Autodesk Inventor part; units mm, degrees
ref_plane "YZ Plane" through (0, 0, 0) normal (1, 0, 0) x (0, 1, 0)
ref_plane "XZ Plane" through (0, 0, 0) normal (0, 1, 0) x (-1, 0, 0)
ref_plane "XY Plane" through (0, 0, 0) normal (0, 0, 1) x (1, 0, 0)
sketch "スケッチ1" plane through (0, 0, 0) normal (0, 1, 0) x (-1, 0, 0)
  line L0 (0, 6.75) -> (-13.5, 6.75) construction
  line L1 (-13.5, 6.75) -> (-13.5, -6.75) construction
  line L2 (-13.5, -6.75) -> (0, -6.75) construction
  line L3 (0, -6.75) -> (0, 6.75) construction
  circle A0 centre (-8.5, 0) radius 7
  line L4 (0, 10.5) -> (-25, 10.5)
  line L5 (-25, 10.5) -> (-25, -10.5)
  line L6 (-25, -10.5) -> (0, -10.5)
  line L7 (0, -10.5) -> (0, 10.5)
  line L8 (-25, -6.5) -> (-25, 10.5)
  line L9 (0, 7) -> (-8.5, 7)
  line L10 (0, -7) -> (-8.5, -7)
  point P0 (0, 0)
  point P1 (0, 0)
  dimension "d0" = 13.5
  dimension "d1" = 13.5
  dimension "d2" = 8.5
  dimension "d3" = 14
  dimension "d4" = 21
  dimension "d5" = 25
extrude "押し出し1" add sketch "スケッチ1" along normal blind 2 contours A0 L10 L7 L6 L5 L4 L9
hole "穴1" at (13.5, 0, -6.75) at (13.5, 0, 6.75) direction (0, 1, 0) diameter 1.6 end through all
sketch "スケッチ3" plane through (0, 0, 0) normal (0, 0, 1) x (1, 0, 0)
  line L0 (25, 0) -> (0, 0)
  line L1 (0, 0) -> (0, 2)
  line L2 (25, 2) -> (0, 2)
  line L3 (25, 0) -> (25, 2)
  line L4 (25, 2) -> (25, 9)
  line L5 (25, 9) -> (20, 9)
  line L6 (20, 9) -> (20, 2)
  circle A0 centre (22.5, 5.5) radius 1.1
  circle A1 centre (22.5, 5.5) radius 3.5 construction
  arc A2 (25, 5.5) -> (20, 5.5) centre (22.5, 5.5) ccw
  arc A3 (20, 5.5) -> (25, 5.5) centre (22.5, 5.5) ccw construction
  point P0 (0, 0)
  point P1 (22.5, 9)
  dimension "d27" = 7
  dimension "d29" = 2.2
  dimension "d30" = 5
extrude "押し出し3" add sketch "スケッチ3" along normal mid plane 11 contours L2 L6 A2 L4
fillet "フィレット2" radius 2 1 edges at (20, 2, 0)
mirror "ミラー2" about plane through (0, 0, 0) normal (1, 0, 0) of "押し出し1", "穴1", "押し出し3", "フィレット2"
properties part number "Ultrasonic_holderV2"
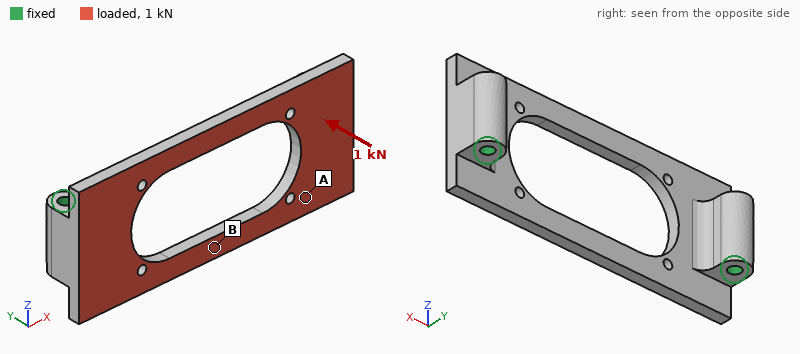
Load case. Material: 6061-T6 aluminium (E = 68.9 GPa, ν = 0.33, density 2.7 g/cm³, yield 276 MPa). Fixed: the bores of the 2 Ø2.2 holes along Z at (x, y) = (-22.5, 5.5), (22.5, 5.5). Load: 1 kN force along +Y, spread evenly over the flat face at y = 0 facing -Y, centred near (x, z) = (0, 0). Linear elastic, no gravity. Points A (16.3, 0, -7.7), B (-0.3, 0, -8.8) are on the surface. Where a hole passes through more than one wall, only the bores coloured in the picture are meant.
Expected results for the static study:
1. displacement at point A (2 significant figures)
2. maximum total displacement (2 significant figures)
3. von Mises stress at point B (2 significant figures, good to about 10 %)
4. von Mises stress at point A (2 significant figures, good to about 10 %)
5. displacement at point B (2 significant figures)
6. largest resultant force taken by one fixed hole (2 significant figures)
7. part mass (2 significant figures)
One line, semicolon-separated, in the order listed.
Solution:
0.042 mm; 0.22 mm; 140 MPa; 75 MPa; 0.21 mm; 530 N; 5.0 g
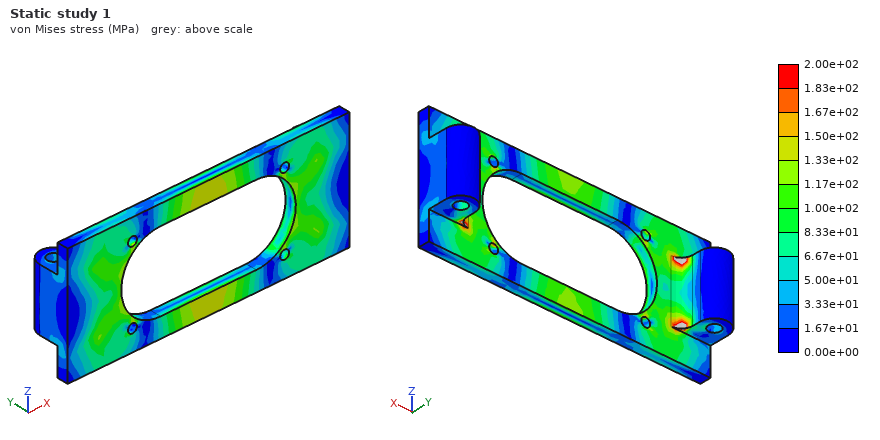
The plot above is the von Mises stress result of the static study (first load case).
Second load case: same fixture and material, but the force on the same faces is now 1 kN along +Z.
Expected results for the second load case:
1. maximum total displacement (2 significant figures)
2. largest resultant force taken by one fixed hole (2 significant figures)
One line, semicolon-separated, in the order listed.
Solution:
40 µm; 500 N
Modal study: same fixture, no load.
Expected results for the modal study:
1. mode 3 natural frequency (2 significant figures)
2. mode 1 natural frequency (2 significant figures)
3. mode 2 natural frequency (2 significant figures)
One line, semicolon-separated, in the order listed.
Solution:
16 kHz; 7000 Hz; 7000 Hz
